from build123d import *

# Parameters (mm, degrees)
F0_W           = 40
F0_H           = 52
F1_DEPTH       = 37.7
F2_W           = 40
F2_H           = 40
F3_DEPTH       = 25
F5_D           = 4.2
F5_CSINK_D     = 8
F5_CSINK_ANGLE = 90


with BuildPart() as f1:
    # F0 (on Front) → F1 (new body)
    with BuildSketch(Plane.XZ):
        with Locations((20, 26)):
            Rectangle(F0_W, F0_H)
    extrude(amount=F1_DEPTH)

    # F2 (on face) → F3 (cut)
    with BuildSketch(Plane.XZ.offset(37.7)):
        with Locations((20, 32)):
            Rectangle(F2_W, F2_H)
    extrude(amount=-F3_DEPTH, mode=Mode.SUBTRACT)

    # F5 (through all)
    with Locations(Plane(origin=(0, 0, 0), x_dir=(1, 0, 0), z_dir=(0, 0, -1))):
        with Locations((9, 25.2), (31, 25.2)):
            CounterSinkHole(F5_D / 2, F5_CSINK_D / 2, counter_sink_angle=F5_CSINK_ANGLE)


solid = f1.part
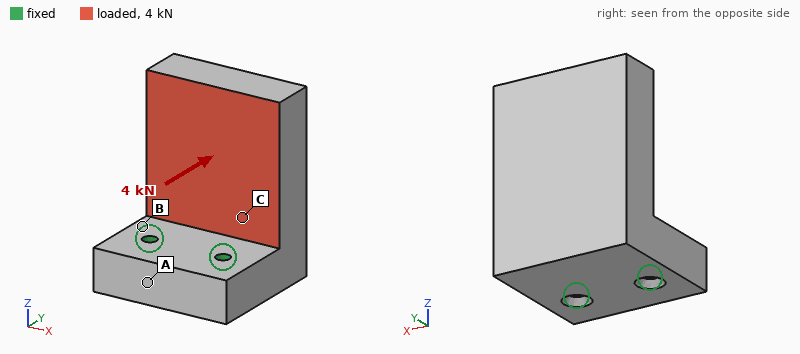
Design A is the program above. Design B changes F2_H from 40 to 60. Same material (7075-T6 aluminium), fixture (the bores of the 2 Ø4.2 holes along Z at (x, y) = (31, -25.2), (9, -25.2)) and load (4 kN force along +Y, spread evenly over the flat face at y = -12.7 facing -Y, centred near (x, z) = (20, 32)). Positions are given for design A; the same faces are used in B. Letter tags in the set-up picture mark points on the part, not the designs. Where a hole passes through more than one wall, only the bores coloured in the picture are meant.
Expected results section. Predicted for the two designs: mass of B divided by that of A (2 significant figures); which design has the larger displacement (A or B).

0.74
B
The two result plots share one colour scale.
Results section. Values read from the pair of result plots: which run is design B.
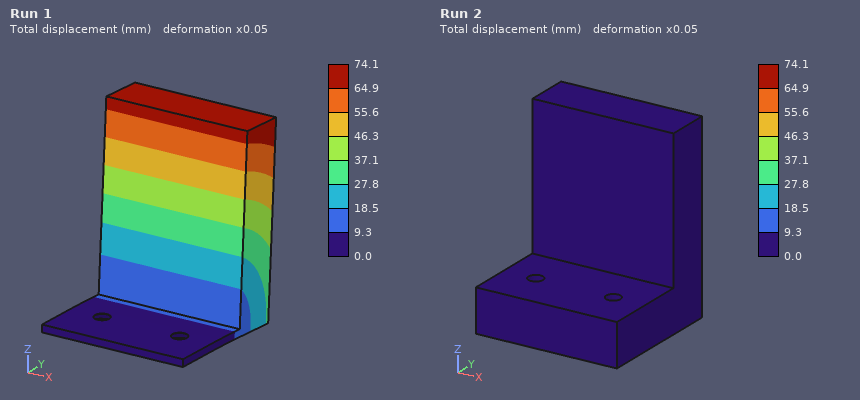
Run 1
